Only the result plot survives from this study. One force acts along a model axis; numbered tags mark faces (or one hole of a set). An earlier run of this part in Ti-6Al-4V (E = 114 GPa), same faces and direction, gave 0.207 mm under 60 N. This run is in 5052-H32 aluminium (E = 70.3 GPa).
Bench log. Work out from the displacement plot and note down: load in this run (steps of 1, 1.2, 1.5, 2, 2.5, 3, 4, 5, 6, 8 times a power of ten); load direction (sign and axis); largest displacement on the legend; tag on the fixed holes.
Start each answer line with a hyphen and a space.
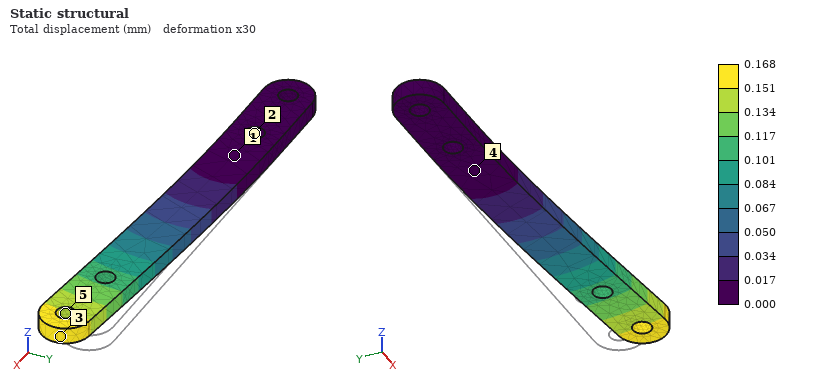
- 30 N
- -Y
- 0.168 mm
- 2
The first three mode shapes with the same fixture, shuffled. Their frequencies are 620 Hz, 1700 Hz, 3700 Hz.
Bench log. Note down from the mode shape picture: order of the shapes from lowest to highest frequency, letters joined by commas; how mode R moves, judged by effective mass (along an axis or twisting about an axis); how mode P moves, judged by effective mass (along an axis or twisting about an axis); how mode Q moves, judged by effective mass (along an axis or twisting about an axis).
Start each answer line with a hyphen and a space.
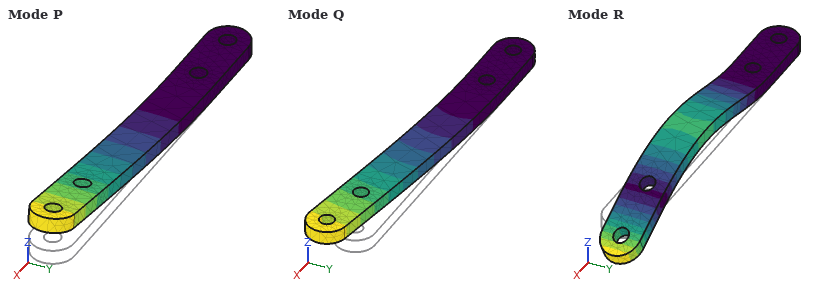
- P, Q, R
- along Z
- along Z
- along Y
